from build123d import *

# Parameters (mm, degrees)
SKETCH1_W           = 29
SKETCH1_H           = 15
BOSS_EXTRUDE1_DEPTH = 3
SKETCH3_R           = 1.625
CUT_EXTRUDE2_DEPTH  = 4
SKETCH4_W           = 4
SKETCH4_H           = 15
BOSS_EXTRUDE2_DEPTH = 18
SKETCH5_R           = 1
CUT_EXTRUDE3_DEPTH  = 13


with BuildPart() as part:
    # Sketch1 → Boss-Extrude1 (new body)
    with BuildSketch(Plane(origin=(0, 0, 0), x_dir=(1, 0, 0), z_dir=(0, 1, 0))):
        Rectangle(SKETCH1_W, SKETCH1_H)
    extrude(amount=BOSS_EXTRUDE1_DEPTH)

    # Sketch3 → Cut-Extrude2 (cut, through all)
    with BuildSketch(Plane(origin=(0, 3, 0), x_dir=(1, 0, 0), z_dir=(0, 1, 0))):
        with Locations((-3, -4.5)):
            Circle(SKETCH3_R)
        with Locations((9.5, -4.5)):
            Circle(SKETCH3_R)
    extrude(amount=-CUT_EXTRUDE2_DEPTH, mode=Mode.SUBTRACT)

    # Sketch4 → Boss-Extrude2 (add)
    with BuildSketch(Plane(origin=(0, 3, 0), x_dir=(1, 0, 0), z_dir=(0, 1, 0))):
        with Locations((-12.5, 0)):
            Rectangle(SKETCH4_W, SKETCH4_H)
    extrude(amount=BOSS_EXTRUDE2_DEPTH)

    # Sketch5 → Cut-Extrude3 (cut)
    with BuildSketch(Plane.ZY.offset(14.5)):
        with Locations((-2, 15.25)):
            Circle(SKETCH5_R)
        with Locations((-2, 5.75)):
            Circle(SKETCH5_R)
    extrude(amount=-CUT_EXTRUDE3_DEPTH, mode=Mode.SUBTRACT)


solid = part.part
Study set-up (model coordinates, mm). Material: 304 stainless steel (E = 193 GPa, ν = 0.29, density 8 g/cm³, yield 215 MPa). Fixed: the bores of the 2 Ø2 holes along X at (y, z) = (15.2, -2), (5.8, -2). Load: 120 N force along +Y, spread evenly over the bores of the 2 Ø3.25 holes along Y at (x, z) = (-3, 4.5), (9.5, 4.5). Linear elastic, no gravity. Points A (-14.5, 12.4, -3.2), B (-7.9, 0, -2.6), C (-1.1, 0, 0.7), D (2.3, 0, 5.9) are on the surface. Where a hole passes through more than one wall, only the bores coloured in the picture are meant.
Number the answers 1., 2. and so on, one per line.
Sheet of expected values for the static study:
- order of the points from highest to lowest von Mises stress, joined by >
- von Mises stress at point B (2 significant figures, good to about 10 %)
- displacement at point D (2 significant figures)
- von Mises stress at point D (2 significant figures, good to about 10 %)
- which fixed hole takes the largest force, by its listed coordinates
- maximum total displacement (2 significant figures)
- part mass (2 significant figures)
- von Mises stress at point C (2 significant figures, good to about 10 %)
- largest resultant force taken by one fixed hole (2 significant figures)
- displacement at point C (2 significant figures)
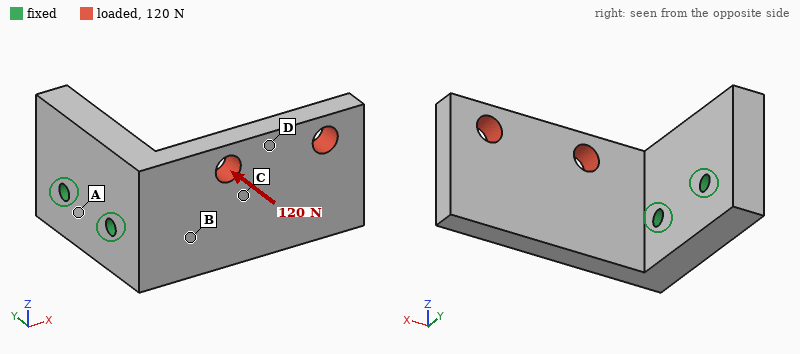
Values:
1. B > C > D > A
2. 59 MPa
3. 33 µm
4. 20 MPa
5. (5.8, -2)
6. 73 µm
7. 18 g
8. 36 MPa
9. 140 N
10. 20 µm
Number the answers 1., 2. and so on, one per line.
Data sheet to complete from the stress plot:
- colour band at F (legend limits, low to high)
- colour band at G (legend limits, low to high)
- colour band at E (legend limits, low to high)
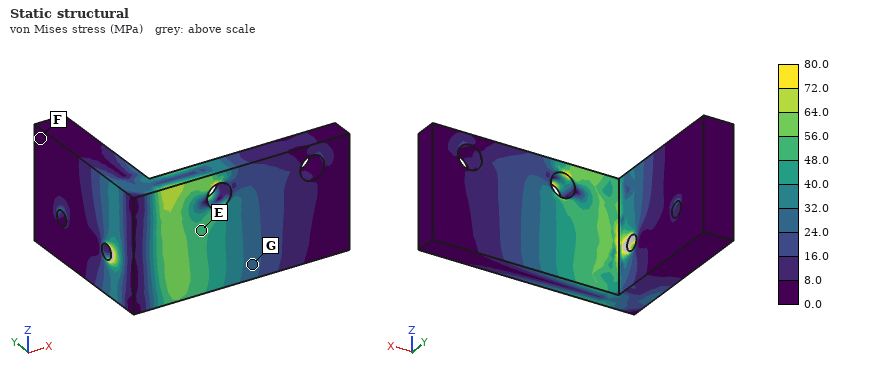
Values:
1. 0.0 to 8.0 MPa
2. 24.0 to 32.0 MPa
3. 48.0 to 56.0 MPa
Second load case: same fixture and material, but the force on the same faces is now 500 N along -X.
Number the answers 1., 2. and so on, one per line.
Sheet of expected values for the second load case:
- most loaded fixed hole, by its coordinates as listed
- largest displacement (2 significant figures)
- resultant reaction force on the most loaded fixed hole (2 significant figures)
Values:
1. (5.8, -2)
2. 34 µm
3. 570 N
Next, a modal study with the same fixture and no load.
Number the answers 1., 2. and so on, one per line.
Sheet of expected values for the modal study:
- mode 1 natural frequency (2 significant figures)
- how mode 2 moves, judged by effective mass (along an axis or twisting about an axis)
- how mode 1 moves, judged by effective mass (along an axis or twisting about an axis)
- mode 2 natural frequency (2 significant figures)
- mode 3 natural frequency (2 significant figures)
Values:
1. 3000 Hz
2. along Z
3. along Y
4. 5800 Hz
5. 12 kHz
